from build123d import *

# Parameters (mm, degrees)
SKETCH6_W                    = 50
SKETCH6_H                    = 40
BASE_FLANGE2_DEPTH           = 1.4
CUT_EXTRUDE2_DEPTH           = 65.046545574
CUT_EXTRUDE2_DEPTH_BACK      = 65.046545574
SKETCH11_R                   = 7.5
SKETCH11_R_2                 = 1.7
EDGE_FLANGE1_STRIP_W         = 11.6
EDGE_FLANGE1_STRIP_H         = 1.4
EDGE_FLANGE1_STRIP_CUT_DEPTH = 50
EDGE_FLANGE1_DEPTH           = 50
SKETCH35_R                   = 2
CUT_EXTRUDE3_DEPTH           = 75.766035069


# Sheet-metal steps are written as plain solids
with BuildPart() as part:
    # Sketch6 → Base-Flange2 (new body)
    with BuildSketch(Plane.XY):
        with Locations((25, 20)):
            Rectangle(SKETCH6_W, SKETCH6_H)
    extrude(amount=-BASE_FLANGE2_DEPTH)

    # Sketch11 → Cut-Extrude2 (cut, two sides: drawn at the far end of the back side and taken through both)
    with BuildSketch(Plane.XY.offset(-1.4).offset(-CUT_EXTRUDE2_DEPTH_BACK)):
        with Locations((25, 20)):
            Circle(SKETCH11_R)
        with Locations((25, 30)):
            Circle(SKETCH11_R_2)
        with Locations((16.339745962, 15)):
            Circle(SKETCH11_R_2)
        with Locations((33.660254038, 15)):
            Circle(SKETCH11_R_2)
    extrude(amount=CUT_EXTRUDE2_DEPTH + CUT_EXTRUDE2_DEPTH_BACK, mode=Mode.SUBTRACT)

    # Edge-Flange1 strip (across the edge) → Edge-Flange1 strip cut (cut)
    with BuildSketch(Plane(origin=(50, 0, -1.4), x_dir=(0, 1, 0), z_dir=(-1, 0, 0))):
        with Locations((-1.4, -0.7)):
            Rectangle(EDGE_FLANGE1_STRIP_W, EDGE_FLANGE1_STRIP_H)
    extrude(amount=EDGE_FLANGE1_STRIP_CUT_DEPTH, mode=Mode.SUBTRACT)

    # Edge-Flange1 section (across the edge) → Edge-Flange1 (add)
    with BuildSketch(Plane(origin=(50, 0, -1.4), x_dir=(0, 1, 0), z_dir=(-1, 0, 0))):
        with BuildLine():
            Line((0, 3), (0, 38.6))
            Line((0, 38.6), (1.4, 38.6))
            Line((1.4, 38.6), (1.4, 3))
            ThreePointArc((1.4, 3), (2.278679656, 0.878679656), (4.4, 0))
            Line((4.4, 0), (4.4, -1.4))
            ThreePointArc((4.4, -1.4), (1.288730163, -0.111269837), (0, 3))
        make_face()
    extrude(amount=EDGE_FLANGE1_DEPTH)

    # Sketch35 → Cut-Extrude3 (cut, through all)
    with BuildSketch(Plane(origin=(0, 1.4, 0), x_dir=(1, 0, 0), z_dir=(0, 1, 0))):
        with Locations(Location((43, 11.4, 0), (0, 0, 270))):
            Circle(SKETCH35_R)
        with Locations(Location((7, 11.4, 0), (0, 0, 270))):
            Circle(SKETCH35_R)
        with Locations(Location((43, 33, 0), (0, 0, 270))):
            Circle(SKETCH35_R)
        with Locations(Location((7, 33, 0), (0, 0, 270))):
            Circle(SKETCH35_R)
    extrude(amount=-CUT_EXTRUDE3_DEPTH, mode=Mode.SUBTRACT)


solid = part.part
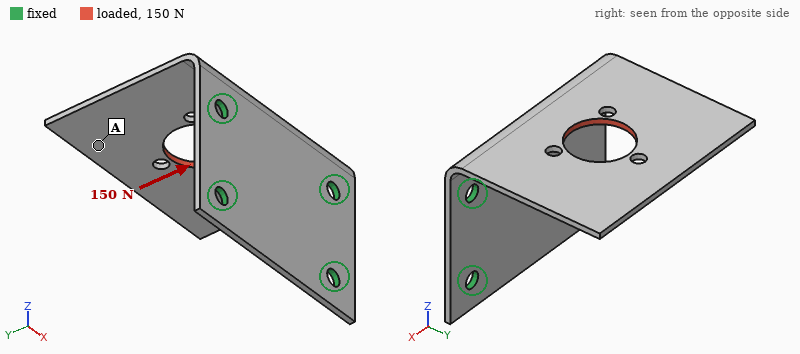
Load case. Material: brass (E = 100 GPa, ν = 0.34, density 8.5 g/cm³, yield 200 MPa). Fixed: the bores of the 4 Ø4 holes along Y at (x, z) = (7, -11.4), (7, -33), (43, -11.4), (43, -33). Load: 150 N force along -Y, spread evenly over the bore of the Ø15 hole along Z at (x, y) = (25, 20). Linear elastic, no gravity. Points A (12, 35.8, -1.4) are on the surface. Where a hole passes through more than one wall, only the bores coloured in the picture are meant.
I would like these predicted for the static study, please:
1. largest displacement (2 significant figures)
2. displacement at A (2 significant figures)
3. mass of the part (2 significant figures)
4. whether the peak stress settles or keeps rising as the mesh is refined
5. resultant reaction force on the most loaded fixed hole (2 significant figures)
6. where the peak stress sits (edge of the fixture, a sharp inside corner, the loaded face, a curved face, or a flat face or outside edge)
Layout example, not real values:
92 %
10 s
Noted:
0.28 mm
0.25 mm
43 g
keeps rising
84 N
edge of the fixture
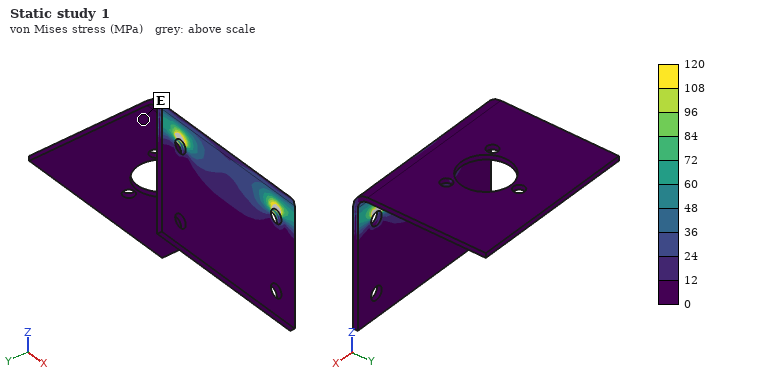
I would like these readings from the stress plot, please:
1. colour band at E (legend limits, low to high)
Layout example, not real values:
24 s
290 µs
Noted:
0 to 12 MPa
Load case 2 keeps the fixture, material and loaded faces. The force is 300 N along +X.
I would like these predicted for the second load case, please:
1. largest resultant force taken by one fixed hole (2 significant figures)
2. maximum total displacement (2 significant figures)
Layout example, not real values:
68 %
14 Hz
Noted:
230 N
0.28 mm
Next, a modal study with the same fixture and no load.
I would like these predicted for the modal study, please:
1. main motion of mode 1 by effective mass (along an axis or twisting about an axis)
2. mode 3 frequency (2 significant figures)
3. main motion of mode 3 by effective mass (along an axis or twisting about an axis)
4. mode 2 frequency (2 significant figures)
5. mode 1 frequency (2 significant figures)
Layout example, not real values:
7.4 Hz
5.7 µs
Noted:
along Z
1600 Hz
along X
820 Hz
370 Hz
